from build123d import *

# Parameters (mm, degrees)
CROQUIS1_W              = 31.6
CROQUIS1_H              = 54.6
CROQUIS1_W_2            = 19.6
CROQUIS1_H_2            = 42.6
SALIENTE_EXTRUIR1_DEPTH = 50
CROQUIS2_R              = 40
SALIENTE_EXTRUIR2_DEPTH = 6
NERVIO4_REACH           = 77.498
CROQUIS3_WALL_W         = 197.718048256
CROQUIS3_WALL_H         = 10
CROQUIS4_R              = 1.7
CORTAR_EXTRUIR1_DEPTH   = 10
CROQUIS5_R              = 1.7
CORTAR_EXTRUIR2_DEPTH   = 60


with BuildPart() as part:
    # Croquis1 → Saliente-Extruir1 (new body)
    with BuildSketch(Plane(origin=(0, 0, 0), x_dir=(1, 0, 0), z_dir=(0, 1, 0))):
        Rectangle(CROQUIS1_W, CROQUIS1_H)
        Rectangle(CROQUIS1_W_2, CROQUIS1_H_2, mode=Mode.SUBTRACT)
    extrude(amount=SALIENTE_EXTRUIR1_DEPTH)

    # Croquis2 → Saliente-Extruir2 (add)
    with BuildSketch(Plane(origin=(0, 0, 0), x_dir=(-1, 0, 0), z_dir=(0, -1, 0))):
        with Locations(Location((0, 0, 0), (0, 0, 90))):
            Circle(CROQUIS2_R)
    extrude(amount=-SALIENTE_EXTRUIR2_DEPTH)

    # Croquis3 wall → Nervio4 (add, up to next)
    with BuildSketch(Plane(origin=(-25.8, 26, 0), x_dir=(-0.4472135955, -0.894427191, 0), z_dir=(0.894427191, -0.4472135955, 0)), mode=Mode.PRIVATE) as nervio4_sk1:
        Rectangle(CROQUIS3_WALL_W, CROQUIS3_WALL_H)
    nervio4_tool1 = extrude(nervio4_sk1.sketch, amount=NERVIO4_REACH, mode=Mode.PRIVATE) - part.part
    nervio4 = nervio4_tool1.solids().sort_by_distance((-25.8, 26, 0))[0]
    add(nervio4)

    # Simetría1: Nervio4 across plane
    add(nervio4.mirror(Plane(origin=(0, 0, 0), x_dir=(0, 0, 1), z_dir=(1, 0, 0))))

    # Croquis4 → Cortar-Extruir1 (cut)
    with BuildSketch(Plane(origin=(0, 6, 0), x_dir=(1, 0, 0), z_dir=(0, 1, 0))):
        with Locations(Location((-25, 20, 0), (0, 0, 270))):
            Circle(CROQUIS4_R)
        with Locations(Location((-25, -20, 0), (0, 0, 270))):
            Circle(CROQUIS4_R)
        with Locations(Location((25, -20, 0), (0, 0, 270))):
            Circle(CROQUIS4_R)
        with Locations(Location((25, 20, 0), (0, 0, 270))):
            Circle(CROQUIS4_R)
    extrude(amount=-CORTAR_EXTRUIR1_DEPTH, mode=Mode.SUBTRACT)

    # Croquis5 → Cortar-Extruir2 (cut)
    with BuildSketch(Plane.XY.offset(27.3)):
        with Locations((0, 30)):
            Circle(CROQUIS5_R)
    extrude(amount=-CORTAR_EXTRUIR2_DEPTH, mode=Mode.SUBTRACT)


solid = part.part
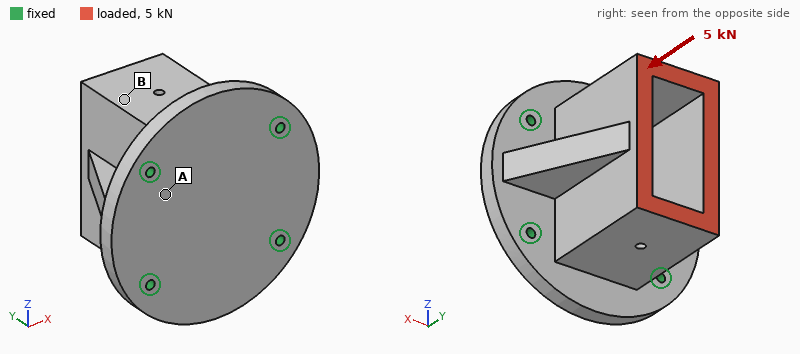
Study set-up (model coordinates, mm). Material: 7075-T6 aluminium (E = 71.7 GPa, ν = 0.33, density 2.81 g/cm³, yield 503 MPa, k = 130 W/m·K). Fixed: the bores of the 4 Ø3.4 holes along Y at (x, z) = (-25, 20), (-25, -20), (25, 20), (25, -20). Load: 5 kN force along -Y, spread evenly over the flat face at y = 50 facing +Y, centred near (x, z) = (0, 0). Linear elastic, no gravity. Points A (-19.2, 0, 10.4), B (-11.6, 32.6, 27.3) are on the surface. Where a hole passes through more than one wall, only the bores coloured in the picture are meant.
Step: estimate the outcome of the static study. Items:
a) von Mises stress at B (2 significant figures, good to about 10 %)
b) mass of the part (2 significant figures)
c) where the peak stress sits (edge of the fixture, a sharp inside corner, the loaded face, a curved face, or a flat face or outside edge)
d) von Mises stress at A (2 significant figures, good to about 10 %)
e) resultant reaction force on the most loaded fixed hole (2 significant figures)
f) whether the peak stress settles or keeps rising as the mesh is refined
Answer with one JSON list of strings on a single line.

["6.3 MPa", "220 g", "edge of the fixture", "11 MPa", "1.3 kN", "keeps rising"]
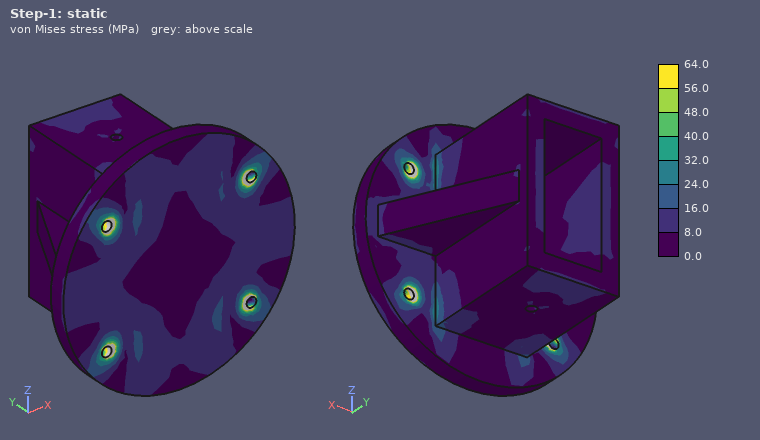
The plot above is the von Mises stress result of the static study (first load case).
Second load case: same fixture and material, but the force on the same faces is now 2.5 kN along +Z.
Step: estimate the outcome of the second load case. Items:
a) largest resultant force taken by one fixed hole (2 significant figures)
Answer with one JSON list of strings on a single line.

["1.6 kN"]
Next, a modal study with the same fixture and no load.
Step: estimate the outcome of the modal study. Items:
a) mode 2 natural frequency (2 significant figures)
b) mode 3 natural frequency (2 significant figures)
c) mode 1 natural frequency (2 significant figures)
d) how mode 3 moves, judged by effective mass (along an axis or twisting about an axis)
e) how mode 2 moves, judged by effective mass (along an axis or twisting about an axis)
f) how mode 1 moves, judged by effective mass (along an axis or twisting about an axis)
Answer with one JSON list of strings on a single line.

["5900 Hz", "7000 Hz", "4700 Hz", "along Y", "along X", "along Z"]
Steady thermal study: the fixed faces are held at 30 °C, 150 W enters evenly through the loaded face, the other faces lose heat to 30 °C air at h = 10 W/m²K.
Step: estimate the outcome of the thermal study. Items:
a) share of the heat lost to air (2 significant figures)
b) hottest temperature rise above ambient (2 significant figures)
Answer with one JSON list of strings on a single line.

["5.6 %", "73 K"]
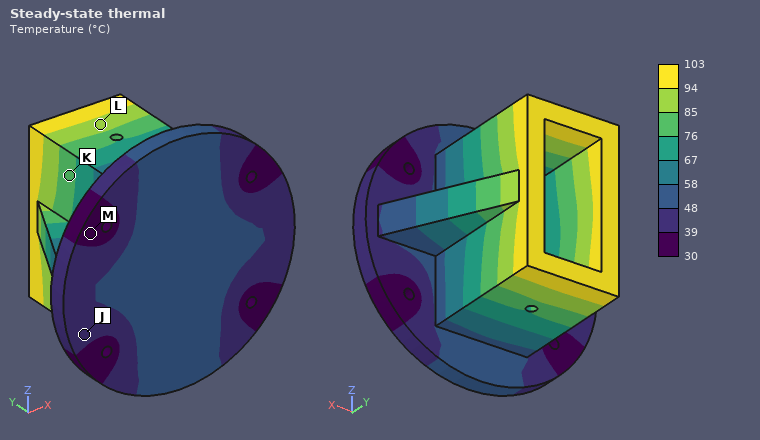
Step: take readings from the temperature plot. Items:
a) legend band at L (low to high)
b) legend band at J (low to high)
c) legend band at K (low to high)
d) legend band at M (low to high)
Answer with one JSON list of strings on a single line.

["85 to 94 °C", "39 to 48 °C", "76 to 85 °C", "30 to 39 °C"]
